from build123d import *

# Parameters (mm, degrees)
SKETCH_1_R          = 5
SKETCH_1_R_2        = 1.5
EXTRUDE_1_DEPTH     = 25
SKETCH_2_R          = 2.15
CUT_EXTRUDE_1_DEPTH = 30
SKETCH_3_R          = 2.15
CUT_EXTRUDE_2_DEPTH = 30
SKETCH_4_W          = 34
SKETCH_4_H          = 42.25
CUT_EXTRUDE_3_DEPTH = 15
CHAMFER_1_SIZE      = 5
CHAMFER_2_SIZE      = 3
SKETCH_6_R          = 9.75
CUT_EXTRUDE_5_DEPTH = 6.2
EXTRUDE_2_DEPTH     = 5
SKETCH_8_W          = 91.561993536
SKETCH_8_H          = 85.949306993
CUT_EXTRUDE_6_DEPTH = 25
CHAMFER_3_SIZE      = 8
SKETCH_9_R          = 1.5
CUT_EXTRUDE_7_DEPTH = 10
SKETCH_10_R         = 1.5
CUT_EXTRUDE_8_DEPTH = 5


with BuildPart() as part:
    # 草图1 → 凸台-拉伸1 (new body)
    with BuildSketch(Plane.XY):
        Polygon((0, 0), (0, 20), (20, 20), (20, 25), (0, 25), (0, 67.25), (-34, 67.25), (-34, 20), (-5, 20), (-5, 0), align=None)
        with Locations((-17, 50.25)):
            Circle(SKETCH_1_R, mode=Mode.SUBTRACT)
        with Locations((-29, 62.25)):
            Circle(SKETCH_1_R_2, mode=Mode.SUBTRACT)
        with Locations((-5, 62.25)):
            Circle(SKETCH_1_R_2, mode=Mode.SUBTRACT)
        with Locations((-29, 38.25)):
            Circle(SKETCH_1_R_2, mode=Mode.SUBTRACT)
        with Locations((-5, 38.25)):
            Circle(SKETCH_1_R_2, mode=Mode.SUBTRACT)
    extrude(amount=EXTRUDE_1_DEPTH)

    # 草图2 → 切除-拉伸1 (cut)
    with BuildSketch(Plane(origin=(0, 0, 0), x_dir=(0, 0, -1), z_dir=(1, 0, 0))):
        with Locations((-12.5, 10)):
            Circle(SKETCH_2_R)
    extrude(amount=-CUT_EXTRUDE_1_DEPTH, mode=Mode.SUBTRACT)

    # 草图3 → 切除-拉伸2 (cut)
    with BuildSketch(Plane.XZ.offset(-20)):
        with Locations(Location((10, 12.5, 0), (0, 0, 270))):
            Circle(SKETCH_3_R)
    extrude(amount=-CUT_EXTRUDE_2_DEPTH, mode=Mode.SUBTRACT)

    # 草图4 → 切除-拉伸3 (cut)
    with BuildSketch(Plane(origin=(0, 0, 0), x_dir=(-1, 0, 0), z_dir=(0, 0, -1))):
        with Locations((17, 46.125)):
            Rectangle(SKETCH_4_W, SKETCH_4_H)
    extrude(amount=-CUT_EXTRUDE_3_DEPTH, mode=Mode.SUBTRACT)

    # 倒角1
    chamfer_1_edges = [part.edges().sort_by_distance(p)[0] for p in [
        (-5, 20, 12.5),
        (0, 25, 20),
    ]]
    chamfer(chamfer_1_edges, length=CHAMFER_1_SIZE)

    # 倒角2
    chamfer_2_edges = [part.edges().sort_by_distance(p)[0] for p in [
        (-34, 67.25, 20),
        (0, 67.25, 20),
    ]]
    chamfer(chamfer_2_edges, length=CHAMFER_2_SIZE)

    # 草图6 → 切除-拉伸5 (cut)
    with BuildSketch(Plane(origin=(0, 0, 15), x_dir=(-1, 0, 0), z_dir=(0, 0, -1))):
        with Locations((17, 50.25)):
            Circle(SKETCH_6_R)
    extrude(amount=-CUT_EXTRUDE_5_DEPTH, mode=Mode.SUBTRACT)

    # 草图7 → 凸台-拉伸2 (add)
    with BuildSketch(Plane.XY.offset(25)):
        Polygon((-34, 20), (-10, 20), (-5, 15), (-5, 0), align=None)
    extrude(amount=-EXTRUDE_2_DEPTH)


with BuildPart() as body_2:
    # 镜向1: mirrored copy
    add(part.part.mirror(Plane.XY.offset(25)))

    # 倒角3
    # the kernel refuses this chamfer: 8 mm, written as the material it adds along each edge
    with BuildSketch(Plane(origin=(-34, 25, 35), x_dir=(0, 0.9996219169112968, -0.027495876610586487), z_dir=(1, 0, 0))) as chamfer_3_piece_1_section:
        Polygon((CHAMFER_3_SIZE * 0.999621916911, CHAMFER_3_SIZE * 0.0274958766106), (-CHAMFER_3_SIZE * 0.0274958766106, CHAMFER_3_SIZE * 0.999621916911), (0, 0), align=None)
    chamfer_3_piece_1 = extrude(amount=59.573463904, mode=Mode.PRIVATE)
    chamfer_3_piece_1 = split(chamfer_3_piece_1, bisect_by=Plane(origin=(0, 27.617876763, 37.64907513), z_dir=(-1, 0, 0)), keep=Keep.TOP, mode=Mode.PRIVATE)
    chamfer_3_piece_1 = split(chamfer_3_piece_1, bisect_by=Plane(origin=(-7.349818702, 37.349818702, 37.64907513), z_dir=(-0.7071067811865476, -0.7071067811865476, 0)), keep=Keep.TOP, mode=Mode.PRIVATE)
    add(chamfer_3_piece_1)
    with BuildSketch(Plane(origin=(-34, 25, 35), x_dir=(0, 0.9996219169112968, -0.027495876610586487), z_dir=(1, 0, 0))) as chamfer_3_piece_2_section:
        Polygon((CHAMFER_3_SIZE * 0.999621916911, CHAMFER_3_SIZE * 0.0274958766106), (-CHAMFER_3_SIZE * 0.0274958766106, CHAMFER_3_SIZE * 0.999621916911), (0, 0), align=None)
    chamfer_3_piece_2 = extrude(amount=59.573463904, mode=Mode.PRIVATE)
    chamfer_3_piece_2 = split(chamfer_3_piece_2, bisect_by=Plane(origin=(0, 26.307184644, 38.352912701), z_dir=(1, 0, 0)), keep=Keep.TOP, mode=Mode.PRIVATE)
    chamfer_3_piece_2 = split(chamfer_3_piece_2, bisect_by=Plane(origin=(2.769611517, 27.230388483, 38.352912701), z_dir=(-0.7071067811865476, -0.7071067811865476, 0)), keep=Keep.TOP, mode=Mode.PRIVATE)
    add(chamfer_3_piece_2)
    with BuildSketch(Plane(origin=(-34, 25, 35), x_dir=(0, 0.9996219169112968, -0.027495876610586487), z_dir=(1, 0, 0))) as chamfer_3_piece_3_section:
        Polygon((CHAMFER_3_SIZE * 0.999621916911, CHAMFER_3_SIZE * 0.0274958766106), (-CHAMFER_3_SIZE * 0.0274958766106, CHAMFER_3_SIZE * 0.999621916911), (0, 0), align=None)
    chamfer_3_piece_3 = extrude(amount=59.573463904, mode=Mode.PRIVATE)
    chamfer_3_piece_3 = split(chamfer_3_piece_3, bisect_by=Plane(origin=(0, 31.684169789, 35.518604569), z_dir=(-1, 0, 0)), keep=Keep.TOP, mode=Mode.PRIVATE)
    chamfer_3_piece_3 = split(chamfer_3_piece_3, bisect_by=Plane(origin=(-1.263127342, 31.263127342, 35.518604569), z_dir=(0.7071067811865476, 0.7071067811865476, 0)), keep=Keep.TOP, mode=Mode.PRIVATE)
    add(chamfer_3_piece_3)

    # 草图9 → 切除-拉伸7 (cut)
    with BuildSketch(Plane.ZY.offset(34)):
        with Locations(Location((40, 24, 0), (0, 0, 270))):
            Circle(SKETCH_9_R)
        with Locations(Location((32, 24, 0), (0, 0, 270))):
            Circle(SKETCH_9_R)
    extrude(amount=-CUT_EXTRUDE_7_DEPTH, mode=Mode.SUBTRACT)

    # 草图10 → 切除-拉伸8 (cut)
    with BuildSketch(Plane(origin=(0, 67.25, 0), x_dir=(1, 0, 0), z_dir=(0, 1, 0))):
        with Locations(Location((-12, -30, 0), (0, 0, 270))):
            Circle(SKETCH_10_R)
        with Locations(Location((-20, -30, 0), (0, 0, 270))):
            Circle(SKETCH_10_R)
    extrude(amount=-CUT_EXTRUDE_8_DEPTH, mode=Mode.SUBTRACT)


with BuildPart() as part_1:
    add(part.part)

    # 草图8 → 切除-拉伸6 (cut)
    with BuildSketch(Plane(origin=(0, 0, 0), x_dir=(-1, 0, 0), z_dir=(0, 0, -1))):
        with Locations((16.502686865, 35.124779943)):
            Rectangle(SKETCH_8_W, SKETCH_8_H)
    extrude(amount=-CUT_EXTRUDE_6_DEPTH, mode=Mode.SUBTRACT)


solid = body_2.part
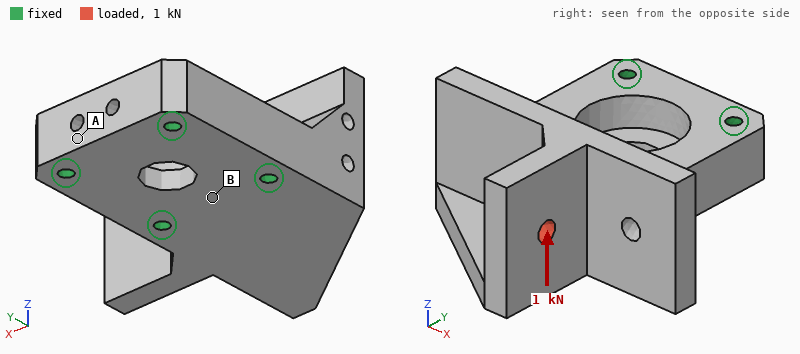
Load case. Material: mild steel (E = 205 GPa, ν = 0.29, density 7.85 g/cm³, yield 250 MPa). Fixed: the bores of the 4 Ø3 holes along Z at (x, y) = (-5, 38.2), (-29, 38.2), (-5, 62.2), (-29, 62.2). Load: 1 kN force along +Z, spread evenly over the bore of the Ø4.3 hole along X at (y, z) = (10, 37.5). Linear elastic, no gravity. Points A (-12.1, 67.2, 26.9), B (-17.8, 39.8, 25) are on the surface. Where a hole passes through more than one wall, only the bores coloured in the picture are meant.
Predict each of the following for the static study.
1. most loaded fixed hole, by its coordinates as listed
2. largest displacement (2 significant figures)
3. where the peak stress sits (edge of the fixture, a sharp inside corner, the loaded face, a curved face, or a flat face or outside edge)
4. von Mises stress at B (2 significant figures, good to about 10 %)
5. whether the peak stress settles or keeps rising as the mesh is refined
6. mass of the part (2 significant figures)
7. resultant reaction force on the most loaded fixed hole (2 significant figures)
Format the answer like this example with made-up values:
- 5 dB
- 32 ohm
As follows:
- (-5, 38.2)
- 31 µm
- edge of the fixture
- 20 MPa
- keeps rising
- 190 g
- 1.1 kN
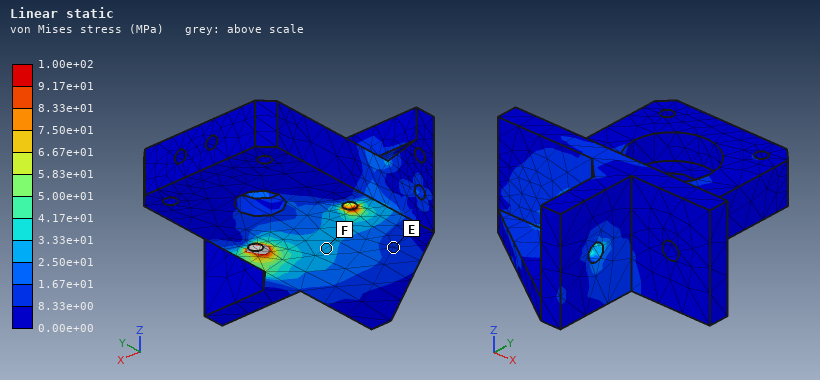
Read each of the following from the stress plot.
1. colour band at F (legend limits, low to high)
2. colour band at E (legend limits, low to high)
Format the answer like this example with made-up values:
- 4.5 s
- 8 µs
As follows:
- 2.50e+01 to 3.33e+01 MPa
- 8.33e+00 to 1.67e+01 MPa
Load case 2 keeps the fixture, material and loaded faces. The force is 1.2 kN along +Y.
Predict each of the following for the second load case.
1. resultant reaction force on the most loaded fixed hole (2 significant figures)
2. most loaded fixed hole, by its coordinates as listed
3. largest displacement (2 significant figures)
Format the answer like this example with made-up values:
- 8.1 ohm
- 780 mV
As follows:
- 1.2 kN
- (-5, 38.2)
- 11 µm
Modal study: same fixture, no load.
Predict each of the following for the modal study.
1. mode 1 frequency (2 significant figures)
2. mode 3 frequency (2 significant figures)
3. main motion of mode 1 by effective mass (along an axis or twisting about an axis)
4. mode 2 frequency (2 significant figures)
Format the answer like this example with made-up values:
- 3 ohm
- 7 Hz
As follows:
- 5000 Hz
- 10 kHz
- along Z
- 9000 Hz
